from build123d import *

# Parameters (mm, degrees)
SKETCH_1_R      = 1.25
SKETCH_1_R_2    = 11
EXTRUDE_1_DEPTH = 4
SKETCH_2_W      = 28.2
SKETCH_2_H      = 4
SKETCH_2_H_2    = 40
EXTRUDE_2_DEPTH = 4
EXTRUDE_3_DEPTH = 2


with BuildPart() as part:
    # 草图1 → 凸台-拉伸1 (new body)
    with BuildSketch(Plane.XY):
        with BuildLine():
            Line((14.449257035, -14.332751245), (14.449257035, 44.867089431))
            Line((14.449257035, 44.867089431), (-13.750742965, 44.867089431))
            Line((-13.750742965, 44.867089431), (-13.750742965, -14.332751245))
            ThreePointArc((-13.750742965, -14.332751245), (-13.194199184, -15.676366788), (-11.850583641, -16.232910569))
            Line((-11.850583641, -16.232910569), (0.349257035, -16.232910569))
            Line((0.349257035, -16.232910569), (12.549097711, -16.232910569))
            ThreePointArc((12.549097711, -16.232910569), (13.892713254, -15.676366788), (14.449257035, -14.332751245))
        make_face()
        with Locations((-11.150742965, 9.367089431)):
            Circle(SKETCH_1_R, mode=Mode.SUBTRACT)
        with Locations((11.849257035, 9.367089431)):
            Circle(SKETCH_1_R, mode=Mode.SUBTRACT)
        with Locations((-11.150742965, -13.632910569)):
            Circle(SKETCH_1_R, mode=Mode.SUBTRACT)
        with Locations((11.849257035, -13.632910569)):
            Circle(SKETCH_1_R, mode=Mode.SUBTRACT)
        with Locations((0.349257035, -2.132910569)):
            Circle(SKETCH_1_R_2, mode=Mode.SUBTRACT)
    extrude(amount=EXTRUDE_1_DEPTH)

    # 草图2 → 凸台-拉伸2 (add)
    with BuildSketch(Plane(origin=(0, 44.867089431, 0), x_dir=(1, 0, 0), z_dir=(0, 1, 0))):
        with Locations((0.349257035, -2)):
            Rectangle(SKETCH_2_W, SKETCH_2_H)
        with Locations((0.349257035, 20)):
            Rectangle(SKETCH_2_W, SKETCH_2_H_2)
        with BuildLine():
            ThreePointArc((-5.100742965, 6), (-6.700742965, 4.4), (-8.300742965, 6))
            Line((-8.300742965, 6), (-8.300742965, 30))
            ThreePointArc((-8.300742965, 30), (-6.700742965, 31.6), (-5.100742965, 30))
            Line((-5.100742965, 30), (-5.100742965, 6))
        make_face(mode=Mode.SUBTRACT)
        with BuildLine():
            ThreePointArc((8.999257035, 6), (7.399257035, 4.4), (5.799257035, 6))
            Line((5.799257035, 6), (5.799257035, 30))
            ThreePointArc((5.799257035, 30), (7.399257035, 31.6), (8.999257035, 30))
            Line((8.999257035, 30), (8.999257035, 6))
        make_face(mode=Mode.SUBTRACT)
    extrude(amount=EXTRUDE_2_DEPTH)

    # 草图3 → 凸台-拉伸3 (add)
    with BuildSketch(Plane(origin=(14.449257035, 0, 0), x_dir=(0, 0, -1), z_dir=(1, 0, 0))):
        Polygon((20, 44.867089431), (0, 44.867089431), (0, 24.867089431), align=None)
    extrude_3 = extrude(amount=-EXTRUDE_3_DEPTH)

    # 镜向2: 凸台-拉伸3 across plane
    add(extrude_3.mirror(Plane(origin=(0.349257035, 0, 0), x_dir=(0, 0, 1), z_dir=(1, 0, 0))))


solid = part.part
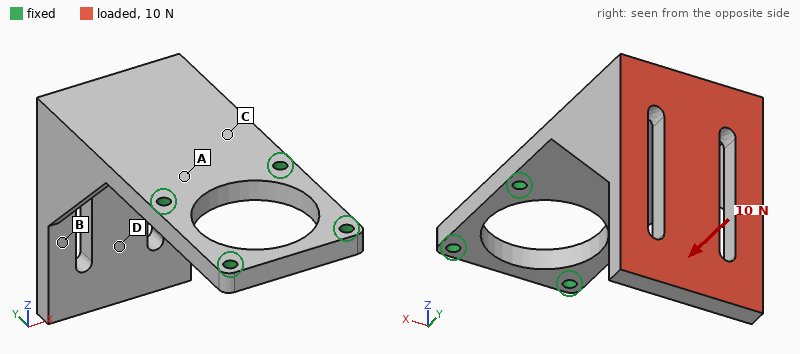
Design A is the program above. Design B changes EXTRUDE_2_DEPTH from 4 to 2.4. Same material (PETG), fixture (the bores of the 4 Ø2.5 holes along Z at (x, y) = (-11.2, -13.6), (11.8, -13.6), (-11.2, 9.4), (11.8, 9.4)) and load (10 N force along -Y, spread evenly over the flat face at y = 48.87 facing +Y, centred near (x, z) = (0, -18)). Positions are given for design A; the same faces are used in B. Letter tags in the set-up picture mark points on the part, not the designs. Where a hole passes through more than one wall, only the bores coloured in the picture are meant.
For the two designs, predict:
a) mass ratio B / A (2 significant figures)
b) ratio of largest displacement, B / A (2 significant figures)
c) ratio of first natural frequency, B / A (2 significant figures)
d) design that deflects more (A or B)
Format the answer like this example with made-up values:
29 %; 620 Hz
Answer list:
0.83; 1.2; 1.2; B
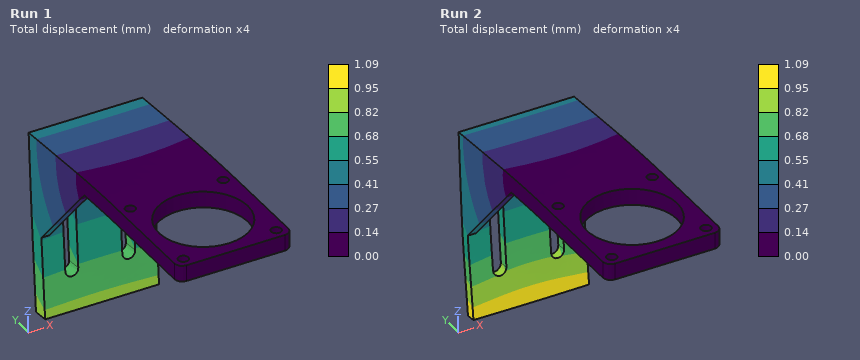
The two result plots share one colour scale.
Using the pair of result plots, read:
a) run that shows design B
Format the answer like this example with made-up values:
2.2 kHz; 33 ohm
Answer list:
Run 2
